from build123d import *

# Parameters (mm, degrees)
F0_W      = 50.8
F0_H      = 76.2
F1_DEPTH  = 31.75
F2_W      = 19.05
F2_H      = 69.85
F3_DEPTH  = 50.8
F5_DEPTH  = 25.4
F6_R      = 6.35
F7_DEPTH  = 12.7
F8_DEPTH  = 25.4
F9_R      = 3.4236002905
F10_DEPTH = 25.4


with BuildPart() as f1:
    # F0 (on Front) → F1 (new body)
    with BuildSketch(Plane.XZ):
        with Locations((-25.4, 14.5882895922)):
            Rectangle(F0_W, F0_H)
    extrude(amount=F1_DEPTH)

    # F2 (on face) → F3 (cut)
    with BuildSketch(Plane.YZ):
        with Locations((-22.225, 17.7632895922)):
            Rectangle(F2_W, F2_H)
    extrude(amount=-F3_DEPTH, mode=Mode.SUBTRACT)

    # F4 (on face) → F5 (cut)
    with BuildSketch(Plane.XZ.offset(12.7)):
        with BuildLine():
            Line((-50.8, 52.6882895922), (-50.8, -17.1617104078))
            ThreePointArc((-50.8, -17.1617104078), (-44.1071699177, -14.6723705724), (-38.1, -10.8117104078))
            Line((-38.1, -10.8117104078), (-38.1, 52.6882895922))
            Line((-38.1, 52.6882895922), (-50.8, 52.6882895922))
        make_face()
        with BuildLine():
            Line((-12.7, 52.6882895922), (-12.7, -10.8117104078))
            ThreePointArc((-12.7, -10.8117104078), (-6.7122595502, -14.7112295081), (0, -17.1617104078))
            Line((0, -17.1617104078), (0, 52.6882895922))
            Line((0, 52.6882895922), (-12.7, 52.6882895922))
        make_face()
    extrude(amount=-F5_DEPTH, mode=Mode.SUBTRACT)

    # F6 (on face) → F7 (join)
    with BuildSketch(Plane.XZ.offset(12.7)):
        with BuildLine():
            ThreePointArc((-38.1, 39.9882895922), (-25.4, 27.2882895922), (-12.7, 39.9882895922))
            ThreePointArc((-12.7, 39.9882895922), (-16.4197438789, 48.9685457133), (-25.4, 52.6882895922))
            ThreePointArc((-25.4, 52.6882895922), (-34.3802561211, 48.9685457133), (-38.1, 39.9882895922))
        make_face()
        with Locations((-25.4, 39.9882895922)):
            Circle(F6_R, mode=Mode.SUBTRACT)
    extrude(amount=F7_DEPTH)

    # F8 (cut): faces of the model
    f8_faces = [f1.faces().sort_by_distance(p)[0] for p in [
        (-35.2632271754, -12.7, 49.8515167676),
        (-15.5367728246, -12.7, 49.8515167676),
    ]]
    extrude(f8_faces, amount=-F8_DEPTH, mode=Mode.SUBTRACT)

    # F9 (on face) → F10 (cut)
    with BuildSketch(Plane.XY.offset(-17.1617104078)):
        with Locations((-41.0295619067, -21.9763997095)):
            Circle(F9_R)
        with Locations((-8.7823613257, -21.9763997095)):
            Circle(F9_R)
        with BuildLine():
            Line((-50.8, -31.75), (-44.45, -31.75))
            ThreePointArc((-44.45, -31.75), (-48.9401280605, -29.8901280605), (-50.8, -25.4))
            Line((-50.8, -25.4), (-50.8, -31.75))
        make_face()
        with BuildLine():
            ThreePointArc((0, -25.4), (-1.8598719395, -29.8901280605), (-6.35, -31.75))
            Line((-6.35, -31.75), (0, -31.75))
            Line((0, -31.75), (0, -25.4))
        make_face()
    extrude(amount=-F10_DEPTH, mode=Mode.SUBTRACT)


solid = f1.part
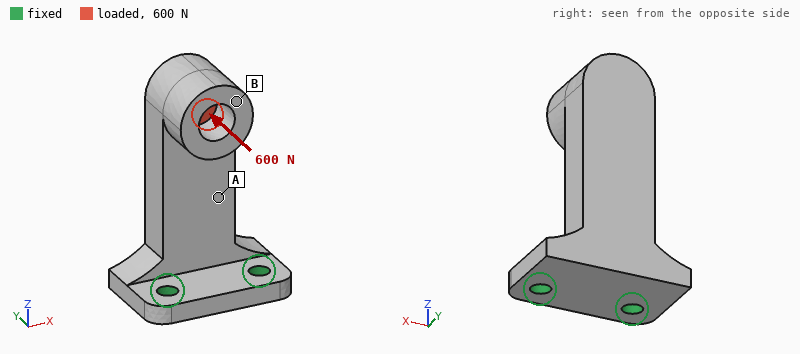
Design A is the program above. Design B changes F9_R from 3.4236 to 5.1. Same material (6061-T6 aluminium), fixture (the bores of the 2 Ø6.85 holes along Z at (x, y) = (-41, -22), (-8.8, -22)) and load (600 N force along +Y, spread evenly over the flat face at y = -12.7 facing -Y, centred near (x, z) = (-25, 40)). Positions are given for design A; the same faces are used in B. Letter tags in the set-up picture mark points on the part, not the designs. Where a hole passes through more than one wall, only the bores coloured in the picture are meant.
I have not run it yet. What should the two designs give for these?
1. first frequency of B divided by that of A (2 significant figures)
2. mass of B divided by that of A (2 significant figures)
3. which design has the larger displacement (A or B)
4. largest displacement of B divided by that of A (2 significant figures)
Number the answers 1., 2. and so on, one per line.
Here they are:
1. 1.1
2. 0.98
3. A
4. 0.87
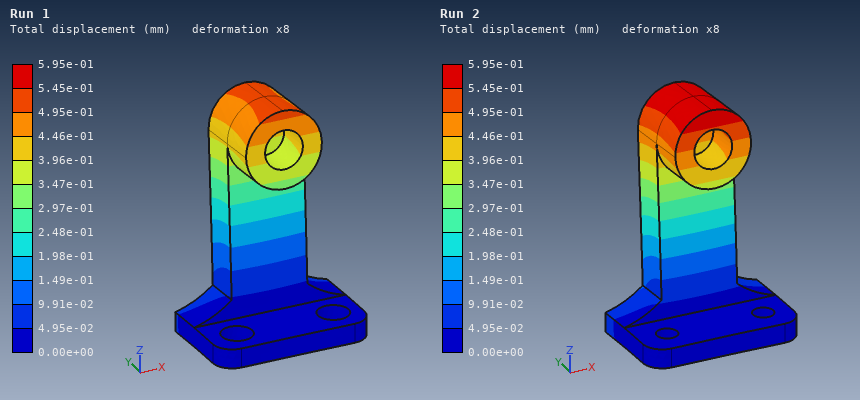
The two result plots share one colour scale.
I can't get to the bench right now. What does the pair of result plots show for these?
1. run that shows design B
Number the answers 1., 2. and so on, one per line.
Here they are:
1. Run 1
